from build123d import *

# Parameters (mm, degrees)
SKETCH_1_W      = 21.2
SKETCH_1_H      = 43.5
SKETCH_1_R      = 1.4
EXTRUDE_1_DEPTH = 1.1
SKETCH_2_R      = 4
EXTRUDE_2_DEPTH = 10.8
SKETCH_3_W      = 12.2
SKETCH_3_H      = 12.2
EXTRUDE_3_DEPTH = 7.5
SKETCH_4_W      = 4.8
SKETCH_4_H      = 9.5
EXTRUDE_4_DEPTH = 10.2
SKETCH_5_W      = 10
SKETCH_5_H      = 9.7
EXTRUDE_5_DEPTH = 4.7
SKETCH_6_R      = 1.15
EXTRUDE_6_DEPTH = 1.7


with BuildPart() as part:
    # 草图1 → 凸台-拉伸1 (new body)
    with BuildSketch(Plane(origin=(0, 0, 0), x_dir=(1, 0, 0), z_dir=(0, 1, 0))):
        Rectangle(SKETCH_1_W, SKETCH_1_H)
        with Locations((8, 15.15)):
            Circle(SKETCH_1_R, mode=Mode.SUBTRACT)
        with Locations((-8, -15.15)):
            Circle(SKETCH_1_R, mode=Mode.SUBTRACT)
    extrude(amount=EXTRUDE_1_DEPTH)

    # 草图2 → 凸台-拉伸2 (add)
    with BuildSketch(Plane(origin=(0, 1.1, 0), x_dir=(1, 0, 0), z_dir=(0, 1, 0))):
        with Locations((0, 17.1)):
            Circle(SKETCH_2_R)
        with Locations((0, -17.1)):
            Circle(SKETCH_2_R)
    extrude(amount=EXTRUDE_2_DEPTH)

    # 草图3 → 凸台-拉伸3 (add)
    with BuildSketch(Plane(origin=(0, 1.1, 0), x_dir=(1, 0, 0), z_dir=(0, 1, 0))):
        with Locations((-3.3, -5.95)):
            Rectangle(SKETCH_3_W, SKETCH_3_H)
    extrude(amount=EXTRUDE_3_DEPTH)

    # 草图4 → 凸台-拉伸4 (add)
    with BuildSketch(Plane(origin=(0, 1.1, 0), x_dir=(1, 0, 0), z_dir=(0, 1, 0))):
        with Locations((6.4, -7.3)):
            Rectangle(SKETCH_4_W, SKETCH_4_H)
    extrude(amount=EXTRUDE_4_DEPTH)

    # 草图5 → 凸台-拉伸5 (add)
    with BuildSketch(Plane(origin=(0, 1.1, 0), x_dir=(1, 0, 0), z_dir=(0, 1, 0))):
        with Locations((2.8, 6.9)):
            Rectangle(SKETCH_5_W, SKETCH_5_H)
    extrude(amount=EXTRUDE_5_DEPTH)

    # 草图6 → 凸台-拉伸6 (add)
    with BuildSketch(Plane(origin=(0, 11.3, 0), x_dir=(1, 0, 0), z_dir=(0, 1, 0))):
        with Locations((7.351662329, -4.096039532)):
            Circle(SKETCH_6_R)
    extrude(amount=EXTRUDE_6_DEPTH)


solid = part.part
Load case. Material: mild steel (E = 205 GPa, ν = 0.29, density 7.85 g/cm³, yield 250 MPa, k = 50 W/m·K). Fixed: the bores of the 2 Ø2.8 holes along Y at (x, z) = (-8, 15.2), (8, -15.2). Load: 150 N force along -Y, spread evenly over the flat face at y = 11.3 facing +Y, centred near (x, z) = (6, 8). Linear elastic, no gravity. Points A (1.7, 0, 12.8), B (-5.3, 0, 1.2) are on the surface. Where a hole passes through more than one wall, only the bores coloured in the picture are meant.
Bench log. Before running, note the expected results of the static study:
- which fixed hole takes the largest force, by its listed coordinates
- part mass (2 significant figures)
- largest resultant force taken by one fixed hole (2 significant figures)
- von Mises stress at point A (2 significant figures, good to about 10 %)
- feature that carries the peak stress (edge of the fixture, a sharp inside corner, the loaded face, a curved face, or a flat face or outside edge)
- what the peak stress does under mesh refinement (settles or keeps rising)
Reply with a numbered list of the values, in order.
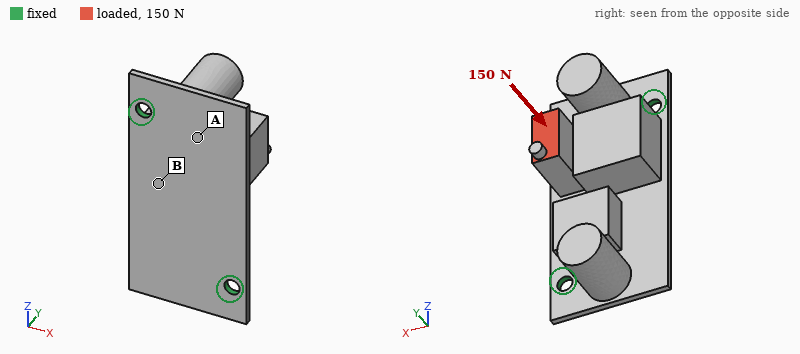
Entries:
1. (-8, 15.2)
2. 32 g
3. 110 N
4. 63 MPa
5. edge of the fixture
6. keeps rising
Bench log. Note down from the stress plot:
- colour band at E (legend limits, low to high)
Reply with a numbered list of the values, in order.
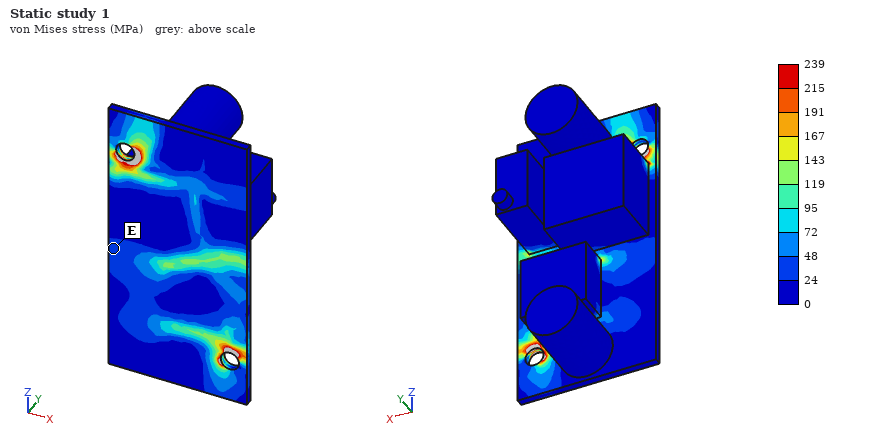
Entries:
1. 24 to 48 MPa
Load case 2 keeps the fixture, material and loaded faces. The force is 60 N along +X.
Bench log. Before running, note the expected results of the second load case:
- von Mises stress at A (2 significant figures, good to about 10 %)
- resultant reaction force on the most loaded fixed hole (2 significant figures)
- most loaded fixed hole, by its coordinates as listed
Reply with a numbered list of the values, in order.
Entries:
1. 38 MPa
2. 43 N
3. (-8, 15.2)
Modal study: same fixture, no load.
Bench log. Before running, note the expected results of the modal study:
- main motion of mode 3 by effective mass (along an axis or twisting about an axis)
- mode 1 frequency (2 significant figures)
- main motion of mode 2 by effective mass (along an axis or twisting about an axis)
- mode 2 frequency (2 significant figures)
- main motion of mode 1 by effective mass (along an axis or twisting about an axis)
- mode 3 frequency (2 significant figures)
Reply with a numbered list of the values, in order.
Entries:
1. along Y
2. 2000 Hz
3. along Y
4. 2900 Hz
5. along X
6. 3700 Hz
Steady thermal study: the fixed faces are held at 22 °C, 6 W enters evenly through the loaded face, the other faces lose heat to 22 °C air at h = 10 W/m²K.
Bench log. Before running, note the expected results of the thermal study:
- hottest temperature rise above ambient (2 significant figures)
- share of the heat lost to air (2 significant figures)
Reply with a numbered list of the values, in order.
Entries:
1. 72 K
2. 13 %
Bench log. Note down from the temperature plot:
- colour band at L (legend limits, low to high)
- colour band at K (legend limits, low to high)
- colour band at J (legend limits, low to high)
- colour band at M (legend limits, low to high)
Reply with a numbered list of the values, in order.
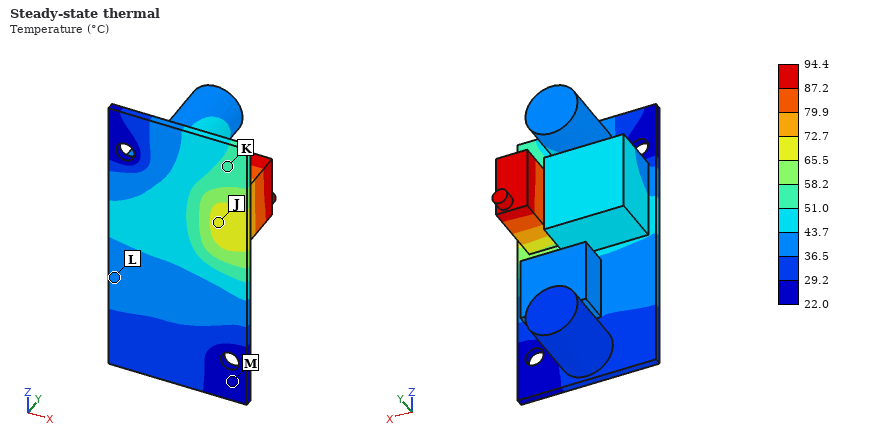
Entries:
1. 36.5 to 43.7 °C
2. 51.0 to 58.2 °C
3. 65.5 to 72.7 °C
4. 22.0 to 29.2 °C
